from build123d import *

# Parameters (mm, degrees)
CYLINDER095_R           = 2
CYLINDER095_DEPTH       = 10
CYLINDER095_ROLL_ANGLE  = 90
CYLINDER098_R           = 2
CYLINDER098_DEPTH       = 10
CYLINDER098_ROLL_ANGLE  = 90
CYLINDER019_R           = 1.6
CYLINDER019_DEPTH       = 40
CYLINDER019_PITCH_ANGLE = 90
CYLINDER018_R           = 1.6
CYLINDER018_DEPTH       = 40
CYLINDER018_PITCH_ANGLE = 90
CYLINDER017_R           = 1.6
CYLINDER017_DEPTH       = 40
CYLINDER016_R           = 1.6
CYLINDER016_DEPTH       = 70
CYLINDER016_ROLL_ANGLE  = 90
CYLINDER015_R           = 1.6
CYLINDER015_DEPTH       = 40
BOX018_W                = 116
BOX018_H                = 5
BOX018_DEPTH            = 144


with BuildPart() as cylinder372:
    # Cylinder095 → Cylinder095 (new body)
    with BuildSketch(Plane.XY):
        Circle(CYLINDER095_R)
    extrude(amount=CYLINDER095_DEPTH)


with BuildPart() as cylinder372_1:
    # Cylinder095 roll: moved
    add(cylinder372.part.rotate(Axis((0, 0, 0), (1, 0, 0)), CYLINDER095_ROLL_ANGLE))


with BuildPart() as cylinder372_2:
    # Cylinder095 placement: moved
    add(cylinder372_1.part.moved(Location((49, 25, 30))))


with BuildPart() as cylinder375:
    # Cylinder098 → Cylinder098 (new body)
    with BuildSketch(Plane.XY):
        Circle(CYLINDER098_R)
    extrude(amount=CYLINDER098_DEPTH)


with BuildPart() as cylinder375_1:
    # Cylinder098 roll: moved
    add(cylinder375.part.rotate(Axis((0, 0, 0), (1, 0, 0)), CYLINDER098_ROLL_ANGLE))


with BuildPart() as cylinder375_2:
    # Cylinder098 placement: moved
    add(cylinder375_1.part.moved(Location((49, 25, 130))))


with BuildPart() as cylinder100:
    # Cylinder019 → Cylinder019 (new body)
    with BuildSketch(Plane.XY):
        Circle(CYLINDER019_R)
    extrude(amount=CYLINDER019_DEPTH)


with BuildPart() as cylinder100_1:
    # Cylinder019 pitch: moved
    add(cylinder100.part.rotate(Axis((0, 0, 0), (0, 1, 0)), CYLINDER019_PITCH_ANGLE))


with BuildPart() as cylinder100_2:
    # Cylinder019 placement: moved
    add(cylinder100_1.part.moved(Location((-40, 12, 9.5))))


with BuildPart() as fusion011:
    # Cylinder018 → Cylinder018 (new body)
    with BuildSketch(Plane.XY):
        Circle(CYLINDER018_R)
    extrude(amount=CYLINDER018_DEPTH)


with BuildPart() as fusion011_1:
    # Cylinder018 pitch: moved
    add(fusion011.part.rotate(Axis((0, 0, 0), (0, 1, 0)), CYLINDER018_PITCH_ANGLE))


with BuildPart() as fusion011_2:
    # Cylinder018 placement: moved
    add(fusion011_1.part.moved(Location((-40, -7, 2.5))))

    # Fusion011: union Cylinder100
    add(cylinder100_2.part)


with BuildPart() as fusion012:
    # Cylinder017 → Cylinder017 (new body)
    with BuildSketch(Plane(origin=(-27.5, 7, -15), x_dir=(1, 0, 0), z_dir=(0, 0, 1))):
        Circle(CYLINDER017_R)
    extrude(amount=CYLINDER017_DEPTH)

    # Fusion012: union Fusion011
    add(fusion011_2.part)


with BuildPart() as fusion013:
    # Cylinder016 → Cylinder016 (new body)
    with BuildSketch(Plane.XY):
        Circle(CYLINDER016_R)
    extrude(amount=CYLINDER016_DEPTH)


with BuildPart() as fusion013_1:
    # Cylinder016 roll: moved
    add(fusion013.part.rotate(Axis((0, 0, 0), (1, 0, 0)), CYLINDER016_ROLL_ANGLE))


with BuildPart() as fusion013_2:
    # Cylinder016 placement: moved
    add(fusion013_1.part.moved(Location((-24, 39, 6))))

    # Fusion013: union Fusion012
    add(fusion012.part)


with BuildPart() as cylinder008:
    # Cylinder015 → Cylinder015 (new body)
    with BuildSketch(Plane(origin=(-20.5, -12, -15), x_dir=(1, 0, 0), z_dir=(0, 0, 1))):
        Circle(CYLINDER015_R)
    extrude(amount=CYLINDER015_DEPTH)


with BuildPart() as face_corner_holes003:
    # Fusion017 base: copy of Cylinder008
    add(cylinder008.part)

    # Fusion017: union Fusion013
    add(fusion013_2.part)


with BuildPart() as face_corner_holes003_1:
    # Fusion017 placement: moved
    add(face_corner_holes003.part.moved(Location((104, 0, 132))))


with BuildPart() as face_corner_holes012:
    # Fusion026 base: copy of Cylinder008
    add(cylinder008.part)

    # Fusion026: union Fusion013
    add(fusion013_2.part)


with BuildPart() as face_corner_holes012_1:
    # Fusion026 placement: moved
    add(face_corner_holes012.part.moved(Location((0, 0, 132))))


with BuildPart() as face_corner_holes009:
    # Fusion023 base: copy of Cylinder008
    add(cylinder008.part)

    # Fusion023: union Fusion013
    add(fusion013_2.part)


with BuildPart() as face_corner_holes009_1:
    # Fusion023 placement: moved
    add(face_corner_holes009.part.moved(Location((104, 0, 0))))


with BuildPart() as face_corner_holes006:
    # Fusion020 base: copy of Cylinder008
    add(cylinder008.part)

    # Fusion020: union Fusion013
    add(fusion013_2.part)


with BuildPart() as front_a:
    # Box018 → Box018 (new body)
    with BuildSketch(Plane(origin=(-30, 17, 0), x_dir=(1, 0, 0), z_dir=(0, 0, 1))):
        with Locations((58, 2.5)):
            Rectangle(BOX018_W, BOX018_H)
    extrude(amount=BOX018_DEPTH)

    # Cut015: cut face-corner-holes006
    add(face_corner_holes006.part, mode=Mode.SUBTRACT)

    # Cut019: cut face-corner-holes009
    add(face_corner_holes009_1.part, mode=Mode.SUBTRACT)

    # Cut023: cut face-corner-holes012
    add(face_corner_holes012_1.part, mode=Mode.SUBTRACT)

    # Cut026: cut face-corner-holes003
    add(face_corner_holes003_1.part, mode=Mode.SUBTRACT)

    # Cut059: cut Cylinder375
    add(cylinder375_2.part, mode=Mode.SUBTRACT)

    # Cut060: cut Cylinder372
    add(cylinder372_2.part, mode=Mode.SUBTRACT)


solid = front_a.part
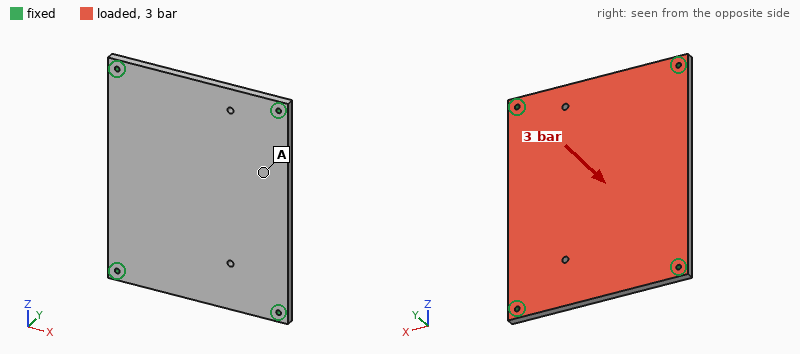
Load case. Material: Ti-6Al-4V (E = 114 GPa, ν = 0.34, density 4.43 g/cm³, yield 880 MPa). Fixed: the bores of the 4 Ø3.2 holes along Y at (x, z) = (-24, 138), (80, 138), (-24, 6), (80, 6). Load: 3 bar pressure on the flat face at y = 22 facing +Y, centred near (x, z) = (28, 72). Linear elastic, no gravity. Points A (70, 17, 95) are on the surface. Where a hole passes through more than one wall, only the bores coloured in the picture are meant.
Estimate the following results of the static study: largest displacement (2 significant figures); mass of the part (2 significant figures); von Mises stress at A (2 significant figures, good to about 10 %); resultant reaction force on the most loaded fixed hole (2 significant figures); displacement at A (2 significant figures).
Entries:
0.46 mm
370 g
58 MPa
1.2 kN
0.32 mm
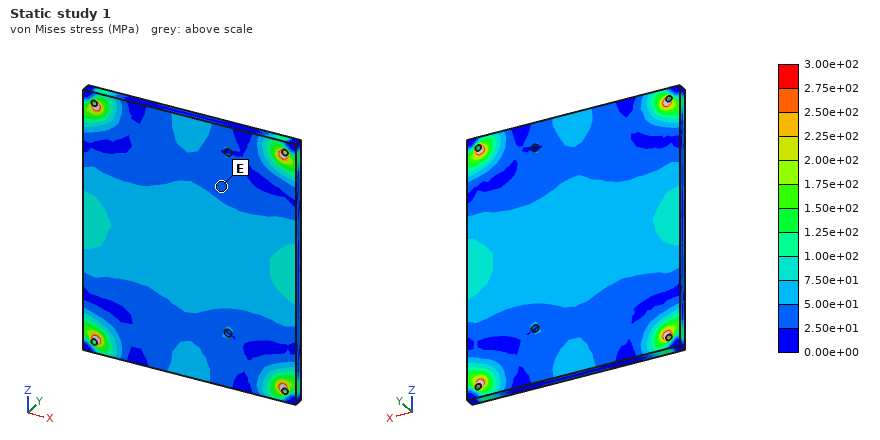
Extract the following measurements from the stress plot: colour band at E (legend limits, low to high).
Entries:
2.50e+01 to 5.00e+01 MPa
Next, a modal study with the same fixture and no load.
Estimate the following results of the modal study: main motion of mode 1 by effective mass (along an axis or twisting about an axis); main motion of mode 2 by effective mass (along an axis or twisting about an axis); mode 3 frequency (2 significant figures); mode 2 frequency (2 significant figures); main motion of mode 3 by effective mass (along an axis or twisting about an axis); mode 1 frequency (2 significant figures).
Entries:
along Y
twisting about Z
2200 Hz
1700 Hz
twisting about X
1000 Hz
